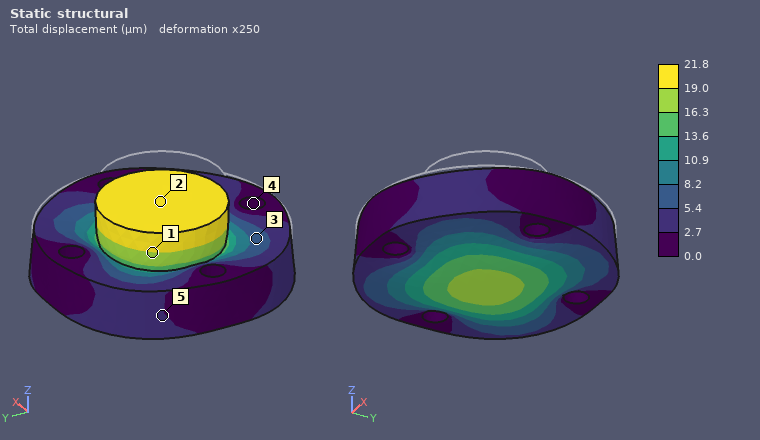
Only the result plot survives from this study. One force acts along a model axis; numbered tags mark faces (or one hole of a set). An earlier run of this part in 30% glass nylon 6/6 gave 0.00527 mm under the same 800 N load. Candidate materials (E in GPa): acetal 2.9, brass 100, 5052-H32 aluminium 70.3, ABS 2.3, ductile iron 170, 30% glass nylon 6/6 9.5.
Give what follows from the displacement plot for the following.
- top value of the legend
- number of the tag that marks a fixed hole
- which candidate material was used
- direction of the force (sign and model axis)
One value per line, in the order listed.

21.8 µm
4
ABS
-Z
